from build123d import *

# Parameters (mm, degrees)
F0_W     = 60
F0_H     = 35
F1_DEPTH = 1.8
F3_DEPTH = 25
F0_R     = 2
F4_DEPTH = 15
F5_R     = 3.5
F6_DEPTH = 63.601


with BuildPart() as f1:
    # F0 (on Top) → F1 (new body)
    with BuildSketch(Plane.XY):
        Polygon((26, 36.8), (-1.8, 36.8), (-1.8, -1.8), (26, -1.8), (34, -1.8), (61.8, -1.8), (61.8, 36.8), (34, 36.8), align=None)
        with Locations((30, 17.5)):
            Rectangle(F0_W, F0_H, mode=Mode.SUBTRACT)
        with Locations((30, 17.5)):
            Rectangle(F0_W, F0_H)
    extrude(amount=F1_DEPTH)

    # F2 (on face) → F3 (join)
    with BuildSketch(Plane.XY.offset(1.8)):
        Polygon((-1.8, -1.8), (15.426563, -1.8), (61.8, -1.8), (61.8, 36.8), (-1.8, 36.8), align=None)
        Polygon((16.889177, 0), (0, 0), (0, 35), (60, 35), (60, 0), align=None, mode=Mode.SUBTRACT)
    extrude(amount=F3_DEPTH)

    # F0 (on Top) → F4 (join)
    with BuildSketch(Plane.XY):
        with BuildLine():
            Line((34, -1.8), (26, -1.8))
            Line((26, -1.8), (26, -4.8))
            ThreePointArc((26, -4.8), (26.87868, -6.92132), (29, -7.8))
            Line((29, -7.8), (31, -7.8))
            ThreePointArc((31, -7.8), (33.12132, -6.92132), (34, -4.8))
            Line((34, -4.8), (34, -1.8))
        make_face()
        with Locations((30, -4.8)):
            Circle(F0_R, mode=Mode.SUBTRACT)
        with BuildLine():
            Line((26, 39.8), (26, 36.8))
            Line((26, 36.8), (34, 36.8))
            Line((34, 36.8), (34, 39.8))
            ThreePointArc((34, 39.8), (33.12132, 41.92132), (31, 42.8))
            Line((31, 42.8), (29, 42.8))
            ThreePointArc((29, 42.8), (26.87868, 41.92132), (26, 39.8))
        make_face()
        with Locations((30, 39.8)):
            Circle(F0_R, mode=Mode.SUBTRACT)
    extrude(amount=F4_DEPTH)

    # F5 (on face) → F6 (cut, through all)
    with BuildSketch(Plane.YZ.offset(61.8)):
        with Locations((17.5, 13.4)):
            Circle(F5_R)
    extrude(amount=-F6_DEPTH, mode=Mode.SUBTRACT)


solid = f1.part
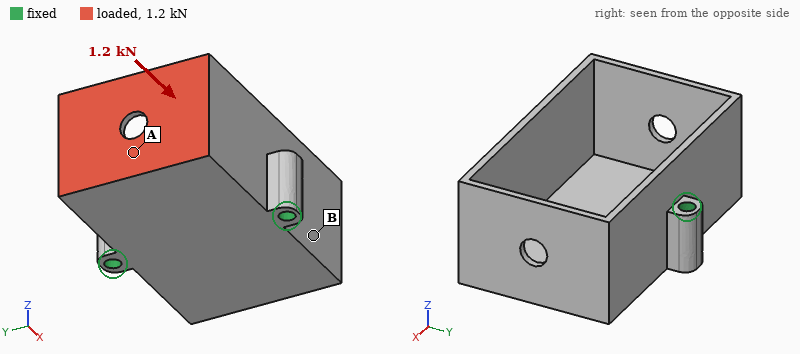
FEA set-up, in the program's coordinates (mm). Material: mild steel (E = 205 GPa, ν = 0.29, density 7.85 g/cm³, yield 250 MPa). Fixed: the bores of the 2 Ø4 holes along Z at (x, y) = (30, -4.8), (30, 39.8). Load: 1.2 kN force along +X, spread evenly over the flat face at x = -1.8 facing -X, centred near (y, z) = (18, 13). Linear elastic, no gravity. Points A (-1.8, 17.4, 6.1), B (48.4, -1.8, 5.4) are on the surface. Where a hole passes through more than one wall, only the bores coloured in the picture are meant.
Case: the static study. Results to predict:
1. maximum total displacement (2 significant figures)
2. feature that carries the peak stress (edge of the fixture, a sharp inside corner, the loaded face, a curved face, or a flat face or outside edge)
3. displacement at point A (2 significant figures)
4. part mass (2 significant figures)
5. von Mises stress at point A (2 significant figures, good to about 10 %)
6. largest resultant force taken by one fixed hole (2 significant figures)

97 µm
the loaded face
22 µm
110 g
47 MPa
600 N
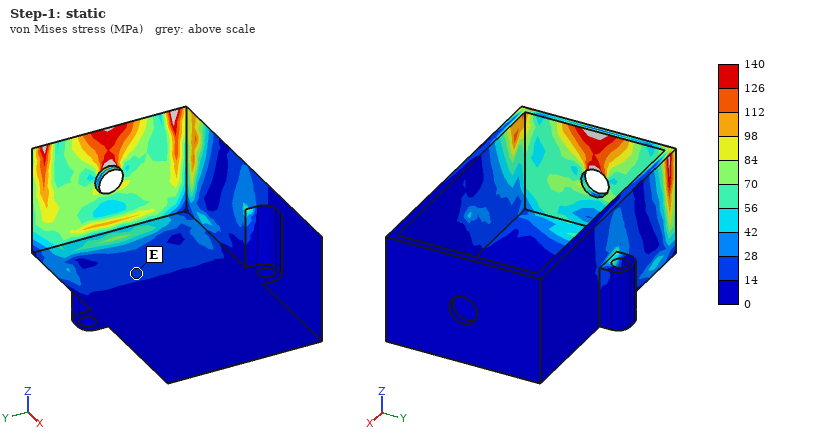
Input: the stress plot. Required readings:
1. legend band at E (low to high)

14 to 28 MPa
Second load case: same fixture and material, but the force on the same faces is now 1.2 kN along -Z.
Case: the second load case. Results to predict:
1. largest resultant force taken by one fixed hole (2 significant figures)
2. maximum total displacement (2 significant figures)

600 N
38 µm
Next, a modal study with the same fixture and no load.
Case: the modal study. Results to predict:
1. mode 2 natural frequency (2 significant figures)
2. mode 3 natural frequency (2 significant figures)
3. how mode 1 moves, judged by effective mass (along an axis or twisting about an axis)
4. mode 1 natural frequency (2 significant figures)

5100 Hz
5800 Hz
twisting about Z
4500 Hz
